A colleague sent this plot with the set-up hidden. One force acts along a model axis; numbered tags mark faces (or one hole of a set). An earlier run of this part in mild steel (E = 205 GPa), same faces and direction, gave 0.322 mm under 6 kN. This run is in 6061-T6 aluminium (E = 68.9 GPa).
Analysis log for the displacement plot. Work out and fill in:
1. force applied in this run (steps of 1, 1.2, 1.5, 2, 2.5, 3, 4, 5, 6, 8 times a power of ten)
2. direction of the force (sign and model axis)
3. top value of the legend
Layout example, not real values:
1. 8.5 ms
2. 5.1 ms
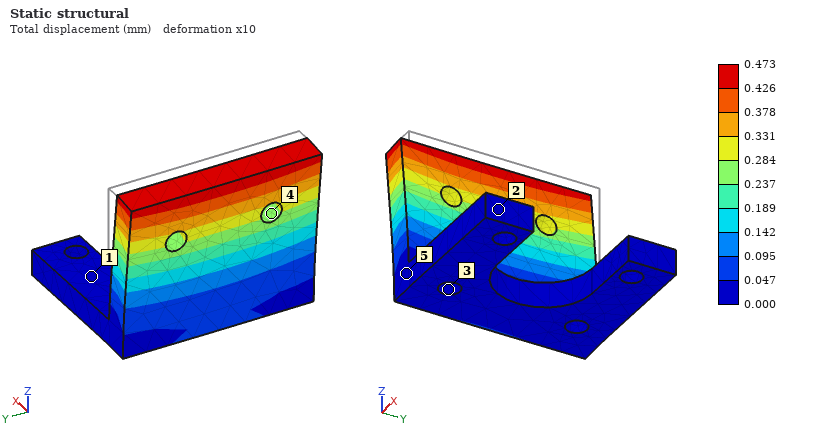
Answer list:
1. 3 kN
2. -X
3. 0.473 mm
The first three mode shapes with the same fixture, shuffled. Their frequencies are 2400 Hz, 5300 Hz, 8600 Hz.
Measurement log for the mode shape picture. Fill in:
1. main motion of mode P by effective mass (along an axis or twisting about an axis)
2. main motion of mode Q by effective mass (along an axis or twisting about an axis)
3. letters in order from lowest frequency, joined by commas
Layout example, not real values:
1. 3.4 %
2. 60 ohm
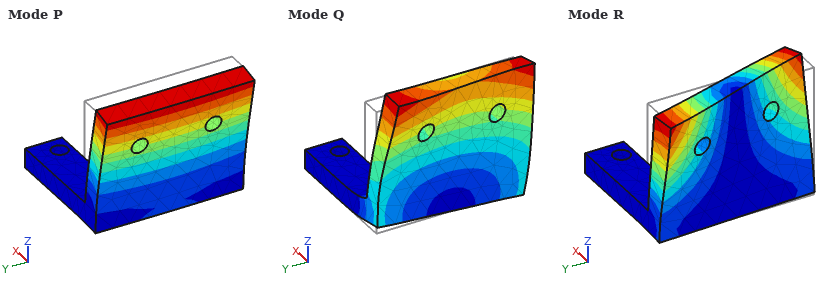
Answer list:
1. along X
2. along Y
3. P, R, Q
